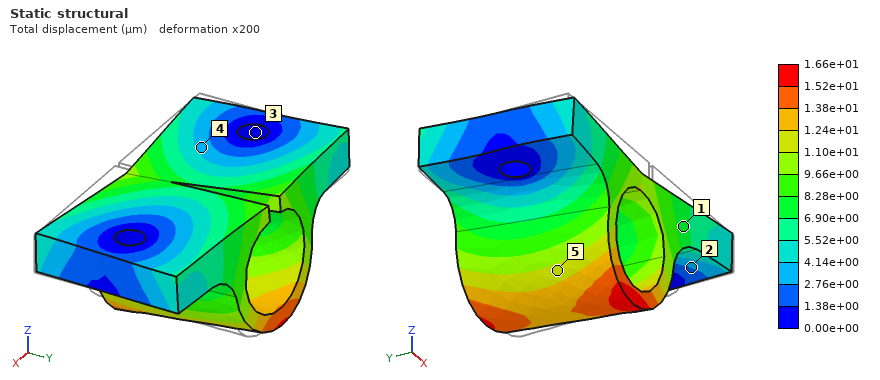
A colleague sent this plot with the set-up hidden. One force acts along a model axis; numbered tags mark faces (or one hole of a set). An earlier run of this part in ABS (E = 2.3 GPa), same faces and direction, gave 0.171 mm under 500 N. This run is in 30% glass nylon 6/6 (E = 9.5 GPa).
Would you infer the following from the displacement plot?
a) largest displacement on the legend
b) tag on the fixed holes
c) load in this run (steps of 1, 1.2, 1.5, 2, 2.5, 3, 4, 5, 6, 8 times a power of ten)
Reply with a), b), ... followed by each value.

a) 1.66e+01 µm
b) 3
c) 200 N
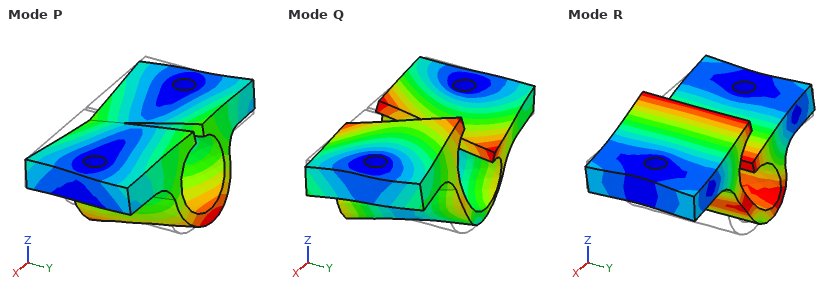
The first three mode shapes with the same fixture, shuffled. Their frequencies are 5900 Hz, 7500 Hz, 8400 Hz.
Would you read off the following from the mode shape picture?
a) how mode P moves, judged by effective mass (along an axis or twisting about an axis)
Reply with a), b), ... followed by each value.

a) along Y
